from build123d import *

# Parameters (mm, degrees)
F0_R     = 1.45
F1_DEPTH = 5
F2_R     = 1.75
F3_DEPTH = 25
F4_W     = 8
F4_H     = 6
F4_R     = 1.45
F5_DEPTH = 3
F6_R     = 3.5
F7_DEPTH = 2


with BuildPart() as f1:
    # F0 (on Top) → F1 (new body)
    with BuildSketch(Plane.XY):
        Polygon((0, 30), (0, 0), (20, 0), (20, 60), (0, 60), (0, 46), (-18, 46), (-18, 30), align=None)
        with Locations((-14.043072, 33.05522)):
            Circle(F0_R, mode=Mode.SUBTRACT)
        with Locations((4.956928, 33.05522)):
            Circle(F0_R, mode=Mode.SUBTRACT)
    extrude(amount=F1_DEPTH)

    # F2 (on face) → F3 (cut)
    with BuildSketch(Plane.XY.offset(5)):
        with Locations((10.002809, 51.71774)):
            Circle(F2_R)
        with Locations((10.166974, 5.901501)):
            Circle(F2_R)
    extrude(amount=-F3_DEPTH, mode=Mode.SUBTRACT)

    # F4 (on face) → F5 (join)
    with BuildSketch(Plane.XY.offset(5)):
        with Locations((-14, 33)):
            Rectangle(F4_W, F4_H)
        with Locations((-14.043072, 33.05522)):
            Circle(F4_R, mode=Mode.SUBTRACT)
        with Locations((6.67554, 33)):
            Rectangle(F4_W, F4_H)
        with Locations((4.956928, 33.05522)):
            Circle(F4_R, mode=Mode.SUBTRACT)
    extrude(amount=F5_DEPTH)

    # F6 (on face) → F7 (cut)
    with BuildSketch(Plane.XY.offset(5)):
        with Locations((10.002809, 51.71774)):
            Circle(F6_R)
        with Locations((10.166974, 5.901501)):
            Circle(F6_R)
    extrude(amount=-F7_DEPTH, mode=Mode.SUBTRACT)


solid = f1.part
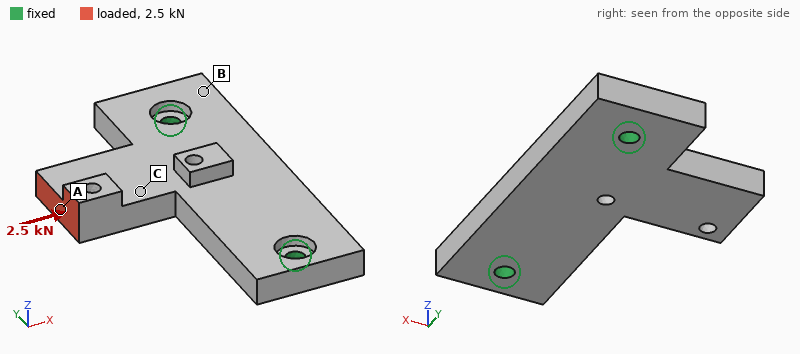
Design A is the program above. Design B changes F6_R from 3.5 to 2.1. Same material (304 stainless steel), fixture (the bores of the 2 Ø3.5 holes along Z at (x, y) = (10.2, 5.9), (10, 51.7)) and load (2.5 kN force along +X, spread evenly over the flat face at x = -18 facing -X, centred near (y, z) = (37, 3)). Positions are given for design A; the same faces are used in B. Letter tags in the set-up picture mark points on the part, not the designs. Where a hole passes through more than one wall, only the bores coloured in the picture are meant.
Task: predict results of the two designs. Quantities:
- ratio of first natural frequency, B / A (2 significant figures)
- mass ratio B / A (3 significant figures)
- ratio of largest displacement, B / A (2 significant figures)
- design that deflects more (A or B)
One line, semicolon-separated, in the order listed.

1.0; 1.01; 0.90; A
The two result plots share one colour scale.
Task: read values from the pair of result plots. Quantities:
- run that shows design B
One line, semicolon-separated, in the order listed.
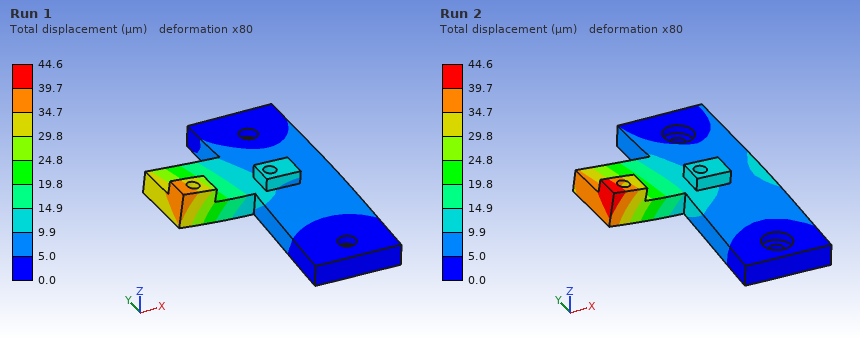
Run 1
